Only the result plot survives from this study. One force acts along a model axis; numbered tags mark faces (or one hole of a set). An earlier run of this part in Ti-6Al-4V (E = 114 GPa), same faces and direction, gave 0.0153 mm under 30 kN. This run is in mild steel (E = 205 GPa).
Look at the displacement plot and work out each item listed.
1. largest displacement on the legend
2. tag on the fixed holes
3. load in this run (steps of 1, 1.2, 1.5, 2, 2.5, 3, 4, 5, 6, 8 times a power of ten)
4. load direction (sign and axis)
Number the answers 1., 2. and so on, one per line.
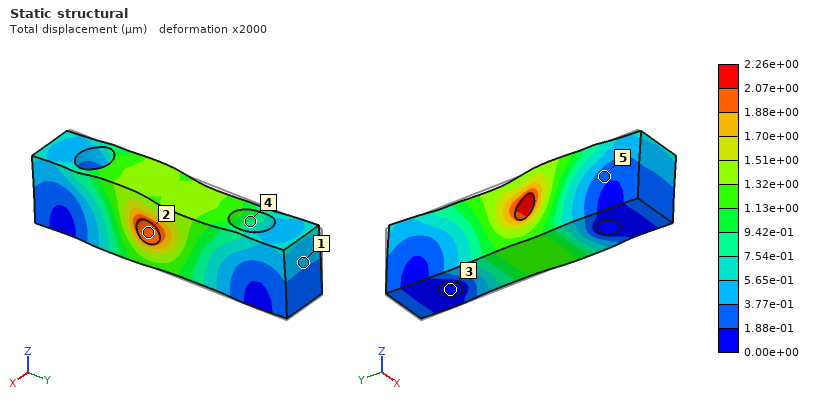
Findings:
1. 2.26e+00 µm
2. 3
3. 8 kN
4. -Y
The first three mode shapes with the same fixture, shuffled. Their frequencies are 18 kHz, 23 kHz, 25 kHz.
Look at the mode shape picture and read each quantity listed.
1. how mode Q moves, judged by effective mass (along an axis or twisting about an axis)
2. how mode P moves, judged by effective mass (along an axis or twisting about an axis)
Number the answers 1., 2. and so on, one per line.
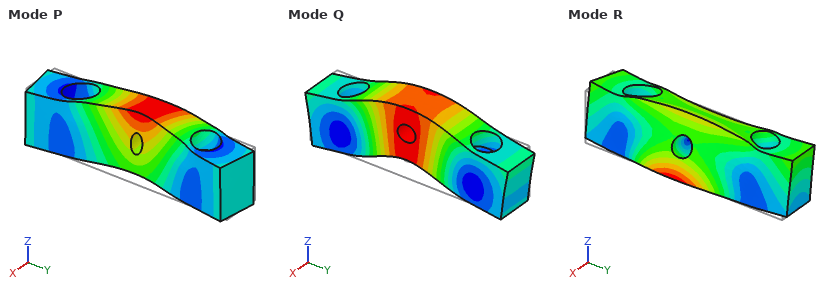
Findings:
1. along Z
2. along X
